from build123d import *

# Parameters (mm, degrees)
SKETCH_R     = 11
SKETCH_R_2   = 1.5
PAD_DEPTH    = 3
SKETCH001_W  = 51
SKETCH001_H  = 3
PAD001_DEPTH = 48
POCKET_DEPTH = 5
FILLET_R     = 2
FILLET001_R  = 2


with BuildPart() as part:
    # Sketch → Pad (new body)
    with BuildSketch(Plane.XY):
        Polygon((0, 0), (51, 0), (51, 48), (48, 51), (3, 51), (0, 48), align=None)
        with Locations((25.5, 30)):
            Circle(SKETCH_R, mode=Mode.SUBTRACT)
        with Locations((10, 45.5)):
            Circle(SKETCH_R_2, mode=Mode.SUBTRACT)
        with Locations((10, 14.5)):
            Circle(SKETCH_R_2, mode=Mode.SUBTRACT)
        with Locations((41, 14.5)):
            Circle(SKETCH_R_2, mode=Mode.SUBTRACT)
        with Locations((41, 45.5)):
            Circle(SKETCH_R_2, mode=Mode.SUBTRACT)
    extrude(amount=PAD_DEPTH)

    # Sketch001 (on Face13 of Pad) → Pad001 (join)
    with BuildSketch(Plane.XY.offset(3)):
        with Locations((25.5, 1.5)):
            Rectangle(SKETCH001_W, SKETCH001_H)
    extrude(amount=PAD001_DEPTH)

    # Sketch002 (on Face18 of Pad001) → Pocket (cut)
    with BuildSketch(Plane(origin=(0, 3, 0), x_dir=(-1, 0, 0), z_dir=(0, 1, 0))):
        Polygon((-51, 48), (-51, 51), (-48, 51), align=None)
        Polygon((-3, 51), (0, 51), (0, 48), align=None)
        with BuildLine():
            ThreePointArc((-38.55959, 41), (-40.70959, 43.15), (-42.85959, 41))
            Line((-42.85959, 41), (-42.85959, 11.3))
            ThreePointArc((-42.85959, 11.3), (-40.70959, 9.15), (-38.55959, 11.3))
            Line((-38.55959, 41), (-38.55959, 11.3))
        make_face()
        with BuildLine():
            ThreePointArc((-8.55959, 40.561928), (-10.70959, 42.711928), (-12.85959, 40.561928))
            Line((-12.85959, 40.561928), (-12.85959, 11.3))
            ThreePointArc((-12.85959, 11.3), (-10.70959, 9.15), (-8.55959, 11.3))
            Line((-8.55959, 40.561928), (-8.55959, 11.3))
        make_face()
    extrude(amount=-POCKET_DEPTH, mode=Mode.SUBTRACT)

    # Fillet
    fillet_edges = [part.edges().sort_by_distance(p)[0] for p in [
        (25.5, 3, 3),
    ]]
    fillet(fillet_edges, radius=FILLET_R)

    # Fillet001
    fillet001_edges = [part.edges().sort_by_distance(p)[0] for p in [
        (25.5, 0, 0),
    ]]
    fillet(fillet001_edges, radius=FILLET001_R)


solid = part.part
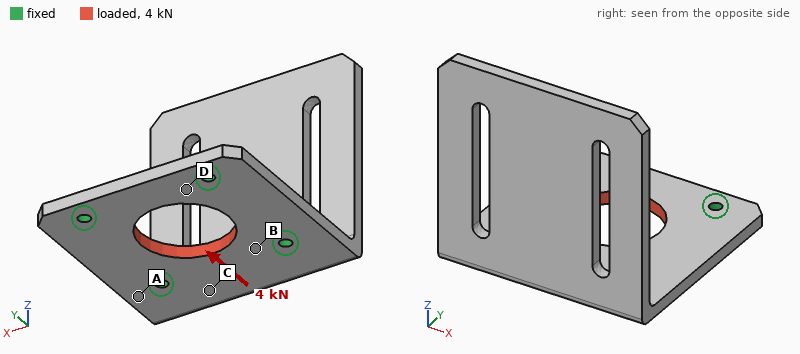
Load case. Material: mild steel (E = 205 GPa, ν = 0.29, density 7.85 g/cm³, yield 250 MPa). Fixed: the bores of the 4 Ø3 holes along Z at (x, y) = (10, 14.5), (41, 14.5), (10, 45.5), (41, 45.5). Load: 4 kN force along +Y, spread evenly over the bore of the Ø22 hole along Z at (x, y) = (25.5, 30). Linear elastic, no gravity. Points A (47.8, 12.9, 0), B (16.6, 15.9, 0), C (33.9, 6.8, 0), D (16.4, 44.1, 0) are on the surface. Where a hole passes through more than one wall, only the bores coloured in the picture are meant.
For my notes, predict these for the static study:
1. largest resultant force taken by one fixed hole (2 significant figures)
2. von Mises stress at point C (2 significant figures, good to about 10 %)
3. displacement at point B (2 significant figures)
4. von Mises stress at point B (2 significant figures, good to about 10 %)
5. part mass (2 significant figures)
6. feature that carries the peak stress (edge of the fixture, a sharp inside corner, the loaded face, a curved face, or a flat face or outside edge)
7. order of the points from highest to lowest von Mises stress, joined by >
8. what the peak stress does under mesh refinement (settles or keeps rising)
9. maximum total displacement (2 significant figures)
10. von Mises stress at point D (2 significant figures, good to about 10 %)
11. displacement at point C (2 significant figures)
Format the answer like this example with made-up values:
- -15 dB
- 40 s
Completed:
- 1.0 kN
- 13 MPa
- 1.3 µm
- 17 MPa
- 100 g
- edge of the fixture
- D > B > C > A
- keeps rising
- 4.1 µm
- 28 MPa
- 1.2 µm
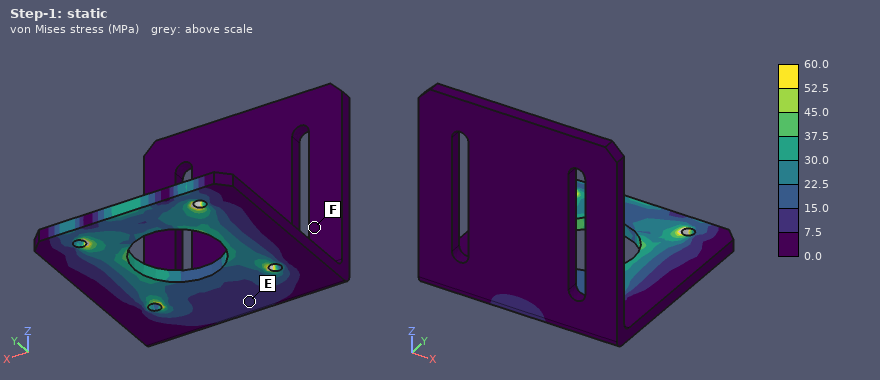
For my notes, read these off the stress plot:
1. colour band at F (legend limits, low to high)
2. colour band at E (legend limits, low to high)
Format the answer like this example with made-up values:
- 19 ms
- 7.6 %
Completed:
- 0.0 to 7.5 MPa
- 7.5 to 15.0 MPa
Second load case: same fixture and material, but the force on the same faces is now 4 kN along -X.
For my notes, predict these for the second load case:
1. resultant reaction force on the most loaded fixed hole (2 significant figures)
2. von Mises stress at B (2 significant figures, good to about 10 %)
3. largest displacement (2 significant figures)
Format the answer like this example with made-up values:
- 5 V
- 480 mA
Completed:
- 1.0 kN
- 26 MPa
- 3.1 µm
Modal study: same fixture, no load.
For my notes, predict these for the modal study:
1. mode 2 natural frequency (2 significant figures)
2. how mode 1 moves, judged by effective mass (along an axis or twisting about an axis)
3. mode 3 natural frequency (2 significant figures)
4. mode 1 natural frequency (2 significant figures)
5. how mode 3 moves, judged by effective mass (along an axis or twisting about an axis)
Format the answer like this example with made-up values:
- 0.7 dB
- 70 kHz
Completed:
- 1900 Hz
- along Y
- 2700 Hz
- 740 Hz
- along X
